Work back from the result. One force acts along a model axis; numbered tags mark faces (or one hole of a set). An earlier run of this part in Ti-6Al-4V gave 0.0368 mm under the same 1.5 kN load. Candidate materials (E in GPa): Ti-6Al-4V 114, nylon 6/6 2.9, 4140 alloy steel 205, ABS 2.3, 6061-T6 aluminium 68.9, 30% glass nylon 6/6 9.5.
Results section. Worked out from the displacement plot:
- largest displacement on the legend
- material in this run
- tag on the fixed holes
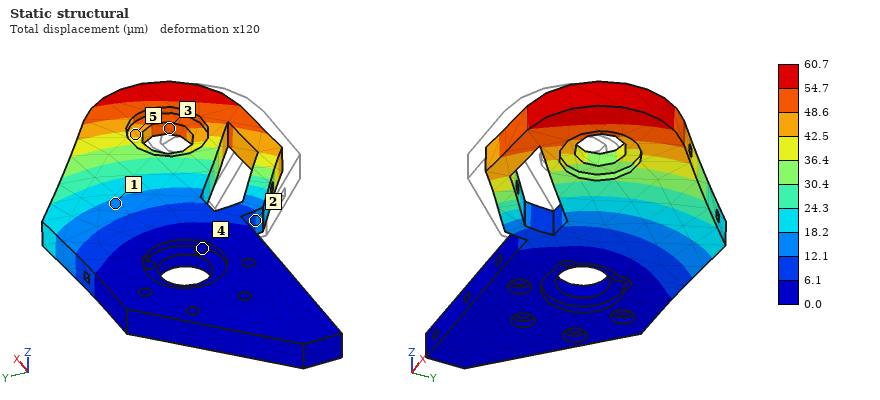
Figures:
60.7 µm
6061-T6 aluminium
4
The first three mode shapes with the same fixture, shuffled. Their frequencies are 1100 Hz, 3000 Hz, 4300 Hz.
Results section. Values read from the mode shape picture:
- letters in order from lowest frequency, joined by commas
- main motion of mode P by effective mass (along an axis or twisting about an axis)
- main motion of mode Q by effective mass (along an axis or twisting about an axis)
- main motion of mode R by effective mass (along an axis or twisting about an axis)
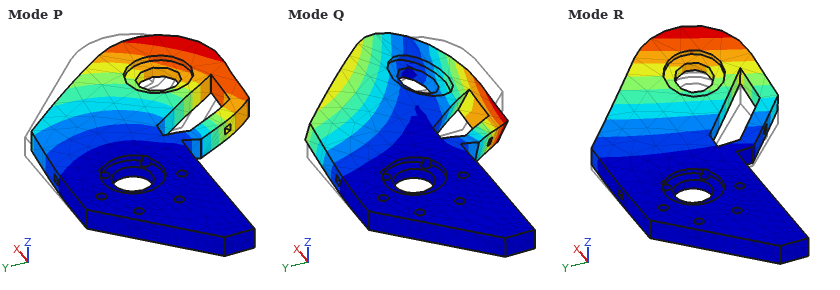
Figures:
R, Q, P
along Y
twisting about X
along Z
